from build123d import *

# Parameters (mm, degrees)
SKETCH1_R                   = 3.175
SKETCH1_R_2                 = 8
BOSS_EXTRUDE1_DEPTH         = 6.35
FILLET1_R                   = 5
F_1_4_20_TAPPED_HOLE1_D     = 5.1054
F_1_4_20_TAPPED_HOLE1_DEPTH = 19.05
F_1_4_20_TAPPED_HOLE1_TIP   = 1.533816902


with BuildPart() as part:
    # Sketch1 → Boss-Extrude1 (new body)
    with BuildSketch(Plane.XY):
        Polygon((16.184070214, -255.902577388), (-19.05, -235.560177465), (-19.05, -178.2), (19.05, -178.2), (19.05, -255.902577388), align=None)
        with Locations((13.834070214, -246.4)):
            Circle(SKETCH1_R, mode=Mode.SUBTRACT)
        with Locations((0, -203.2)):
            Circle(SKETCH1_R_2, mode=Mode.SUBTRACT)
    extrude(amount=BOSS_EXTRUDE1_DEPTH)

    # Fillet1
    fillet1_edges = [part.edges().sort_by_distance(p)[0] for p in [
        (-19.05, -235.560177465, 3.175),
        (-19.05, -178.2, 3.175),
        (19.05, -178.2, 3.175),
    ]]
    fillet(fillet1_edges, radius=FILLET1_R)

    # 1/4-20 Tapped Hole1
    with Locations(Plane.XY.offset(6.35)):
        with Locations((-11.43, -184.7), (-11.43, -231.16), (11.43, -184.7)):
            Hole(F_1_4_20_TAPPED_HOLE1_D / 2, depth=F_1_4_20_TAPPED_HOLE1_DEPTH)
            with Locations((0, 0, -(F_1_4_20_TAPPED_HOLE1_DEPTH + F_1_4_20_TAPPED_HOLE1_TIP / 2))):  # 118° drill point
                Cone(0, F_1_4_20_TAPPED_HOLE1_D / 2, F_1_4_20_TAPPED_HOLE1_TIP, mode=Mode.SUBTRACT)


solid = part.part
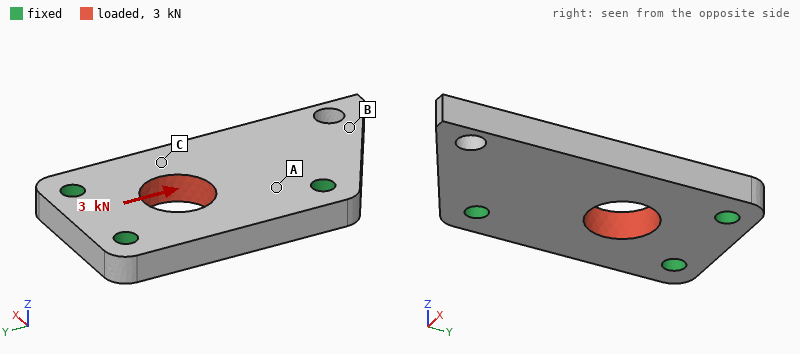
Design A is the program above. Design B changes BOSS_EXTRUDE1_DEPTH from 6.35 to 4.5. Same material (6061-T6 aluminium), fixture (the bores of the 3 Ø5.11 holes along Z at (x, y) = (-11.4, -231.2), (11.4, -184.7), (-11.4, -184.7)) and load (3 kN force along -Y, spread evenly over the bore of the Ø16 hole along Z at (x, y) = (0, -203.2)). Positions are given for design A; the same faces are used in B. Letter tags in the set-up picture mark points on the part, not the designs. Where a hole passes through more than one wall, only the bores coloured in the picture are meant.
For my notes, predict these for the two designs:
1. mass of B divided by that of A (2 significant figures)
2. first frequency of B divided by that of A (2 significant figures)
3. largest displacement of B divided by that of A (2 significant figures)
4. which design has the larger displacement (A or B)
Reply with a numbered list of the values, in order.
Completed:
1. 0.71
2. 0.74
3. 1.4
4. B
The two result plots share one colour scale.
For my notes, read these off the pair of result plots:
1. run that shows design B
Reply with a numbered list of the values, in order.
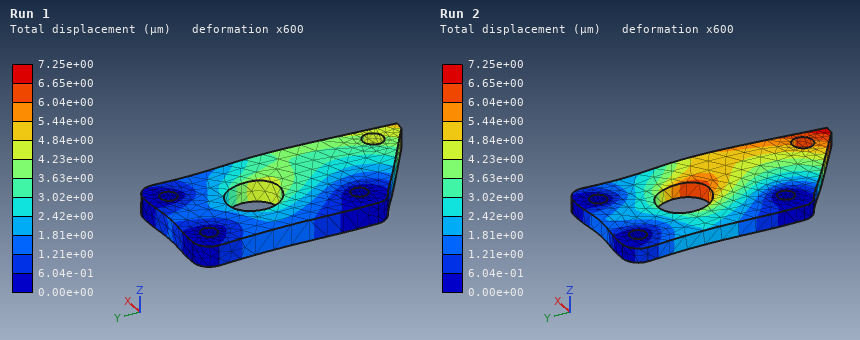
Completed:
1. Run 2
